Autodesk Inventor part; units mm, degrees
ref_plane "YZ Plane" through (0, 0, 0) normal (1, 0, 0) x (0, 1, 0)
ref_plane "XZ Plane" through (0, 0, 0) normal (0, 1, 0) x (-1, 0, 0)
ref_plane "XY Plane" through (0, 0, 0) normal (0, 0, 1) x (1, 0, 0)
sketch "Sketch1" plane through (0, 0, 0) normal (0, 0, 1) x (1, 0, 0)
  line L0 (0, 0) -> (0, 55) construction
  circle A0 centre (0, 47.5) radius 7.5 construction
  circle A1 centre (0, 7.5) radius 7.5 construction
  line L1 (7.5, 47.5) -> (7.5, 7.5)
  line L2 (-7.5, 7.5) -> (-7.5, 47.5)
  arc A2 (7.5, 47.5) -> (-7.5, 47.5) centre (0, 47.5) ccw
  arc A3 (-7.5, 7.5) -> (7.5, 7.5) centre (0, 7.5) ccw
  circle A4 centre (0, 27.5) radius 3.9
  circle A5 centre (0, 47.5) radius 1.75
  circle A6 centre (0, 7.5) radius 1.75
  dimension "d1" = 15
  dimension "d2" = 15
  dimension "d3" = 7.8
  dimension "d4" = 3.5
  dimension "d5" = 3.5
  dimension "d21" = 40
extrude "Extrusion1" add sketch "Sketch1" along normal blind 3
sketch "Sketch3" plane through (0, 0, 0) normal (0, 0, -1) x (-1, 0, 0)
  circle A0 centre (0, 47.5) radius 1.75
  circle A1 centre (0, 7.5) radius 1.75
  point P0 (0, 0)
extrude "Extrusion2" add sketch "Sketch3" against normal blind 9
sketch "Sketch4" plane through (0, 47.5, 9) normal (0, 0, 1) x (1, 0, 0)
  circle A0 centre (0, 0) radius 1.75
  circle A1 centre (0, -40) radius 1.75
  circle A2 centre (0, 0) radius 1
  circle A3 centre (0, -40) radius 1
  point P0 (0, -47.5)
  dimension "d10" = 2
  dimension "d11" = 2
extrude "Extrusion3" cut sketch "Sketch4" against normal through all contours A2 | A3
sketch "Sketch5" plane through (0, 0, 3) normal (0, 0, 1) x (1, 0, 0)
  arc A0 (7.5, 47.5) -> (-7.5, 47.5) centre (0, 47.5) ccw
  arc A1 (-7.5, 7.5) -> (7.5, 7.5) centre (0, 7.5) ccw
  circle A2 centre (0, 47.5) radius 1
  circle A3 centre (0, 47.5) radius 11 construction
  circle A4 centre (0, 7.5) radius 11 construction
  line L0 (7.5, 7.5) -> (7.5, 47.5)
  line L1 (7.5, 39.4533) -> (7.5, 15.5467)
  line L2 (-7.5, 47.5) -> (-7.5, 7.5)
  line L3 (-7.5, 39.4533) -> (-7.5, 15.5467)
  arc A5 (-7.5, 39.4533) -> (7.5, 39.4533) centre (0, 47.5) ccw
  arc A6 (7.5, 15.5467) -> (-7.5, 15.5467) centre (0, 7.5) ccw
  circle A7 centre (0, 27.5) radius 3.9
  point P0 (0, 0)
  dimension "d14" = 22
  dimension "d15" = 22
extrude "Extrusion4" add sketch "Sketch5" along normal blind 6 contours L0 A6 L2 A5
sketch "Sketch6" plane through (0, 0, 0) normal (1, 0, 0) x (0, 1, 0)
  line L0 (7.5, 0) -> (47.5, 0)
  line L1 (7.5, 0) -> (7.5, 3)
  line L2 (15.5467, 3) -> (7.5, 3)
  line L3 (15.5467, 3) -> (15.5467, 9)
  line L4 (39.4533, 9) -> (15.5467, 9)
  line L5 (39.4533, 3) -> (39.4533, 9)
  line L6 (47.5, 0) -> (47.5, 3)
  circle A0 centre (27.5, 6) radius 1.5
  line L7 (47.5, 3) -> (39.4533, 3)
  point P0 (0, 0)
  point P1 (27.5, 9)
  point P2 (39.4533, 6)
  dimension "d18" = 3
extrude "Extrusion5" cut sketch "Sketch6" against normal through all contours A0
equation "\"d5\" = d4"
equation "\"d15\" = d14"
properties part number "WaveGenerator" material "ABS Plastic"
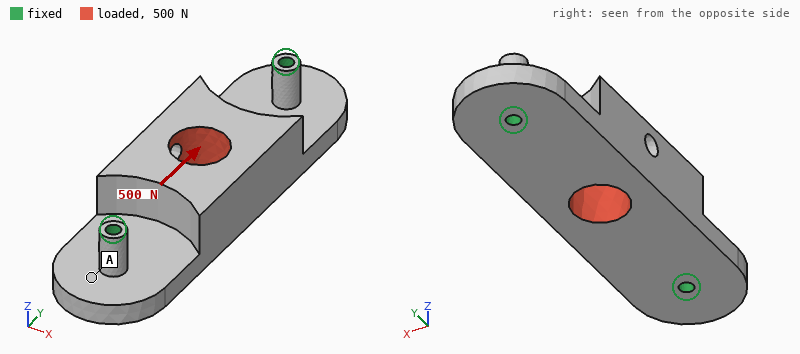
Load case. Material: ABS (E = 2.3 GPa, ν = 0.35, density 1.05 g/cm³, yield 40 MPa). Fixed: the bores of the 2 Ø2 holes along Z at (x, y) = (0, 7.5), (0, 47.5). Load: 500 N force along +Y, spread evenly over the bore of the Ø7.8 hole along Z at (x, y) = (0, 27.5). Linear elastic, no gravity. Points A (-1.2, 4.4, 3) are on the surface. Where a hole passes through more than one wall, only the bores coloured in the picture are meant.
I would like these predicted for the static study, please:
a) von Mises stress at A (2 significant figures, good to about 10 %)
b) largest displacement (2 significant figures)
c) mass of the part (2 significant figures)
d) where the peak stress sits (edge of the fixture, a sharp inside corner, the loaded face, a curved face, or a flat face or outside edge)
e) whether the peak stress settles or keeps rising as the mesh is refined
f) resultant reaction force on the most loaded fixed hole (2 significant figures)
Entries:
2.6 MPa
0.12 mm
3.9 g
edge of the fixture
keeps rising
250 N
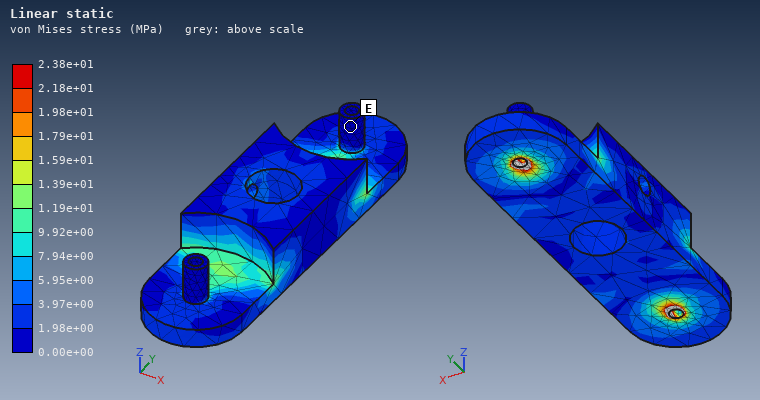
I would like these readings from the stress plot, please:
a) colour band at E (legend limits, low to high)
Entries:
0.00e+00 to 1.98e+00 MPa
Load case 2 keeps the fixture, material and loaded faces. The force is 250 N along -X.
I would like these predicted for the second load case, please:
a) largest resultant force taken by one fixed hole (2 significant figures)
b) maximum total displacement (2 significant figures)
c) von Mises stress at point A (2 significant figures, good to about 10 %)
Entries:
130 N
0.48 mm
4.8 MPa
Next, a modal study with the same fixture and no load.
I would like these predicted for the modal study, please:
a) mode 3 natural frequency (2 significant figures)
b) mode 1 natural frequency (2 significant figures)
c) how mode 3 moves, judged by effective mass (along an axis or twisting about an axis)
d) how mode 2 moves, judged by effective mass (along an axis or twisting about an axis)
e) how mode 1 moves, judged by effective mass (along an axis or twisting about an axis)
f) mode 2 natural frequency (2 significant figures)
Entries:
5300 Hz
2300 Hz
along X
along Z
along X
2700 Hz
